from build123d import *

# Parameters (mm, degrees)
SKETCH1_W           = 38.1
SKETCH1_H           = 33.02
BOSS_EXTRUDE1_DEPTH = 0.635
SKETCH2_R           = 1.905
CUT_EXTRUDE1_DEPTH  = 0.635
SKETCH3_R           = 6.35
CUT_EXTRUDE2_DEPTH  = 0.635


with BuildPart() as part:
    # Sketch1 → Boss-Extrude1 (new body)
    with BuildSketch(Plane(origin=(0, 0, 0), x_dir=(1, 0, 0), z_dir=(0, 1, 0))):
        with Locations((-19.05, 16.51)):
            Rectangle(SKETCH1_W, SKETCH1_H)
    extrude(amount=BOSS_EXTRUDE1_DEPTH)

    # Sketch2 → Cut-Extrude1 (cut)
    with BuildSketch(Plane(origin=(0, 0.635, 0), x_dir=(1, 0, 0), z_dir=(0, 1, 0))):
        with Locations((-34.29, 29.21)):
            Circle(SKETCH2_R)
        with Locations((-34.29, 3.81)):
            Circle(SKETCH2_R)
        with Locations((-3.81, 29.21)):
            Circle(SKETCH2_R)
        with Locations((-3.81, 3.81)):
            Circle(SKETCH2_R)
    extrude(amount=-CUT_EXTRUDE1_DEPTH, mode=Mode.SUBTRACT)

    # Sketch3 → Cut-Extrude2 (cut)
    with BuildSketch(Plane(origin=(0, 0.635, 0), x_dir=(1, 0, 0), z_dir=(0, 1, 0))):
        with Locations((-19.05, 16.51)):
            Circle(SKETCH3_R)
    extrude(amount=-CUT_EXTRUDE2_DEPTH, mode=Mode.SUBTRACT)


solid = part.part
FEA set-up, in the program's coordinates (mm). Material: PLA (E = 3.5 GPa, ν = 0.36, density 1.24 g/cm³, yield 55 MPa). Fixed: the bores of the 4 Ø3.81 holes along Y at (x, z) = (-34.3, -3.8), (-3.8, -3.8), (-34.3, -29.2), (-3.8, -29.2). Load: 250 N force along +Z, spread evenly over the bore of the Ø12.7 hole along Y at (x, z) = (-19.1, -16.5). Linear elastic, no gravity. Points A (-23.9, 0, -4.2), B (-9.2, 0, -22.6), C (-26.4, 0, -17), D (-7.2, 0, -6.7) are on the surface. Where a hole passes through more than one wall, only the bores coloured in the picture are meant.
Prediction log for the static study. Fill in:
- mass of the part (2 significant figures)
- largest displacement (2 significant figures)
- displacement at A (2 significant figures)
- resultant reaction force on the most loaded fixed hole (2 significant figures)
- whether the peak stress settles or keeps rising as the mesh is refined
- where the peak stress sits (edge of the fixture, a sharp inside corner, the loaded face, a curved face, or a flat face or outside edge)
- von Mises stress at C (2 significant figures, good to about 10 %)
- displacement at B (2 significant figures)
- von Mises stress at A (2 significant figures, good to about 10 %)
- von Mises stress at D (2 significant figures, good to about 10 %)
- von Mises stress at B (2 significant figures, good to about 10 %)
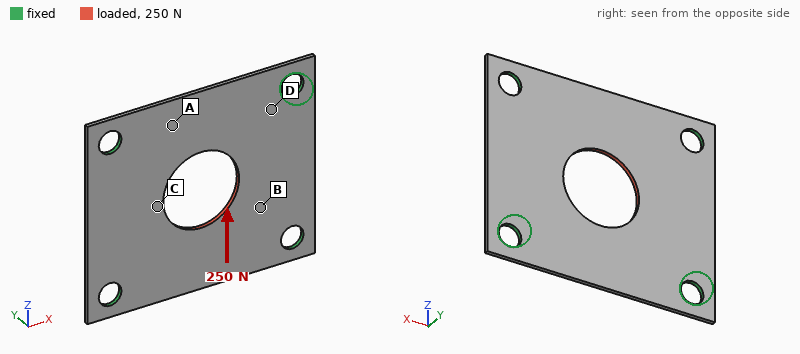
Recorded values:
0.85 g
80 µm
58 µm
71 N
keeps rising
edge of the fixture
17 MPa
33 µm
7.3 MPa
14 MPa
12 MPa
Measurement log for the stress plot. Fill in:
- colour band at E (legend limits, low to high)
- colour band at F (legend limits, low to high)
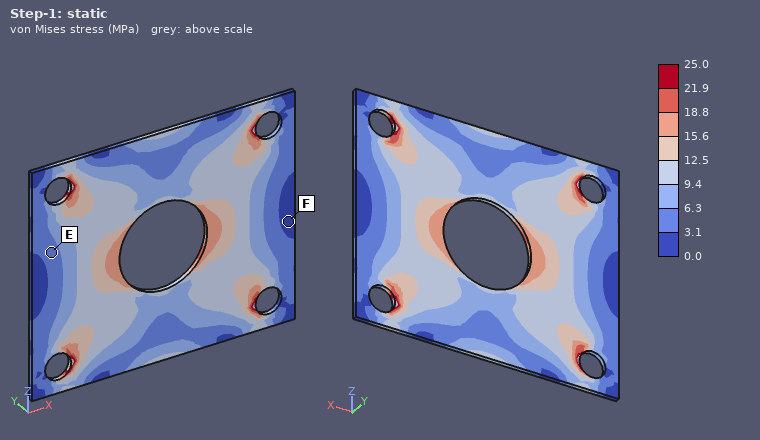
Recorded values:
3.1 to 6.3 MPa
0.0 to 3.1 MPa
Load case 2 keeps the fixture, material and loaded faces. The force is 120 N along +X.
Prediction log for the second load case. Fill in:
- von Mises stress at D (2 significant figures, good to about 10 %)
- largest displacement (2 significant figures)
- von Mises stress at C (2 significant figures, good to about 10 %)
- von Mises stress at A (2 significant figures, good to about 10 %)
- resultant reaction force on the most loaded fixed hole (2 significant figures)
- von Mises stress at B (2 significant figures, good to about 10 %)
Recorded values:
6.7 MPa
27 µm
4.2 MPa
2.6 MPa
32 N
4.9 MPa
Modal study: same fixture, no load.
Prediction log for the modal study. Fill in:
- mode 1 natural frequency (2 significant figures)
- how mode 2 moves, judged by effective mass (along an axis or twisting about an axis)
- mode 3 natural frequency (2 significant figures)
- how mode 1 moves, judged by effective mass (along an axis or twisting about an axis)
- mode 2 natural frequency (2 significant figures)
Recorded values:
1300 Hz
twisting about X
2000 Hz
along Y
1600 Hz
